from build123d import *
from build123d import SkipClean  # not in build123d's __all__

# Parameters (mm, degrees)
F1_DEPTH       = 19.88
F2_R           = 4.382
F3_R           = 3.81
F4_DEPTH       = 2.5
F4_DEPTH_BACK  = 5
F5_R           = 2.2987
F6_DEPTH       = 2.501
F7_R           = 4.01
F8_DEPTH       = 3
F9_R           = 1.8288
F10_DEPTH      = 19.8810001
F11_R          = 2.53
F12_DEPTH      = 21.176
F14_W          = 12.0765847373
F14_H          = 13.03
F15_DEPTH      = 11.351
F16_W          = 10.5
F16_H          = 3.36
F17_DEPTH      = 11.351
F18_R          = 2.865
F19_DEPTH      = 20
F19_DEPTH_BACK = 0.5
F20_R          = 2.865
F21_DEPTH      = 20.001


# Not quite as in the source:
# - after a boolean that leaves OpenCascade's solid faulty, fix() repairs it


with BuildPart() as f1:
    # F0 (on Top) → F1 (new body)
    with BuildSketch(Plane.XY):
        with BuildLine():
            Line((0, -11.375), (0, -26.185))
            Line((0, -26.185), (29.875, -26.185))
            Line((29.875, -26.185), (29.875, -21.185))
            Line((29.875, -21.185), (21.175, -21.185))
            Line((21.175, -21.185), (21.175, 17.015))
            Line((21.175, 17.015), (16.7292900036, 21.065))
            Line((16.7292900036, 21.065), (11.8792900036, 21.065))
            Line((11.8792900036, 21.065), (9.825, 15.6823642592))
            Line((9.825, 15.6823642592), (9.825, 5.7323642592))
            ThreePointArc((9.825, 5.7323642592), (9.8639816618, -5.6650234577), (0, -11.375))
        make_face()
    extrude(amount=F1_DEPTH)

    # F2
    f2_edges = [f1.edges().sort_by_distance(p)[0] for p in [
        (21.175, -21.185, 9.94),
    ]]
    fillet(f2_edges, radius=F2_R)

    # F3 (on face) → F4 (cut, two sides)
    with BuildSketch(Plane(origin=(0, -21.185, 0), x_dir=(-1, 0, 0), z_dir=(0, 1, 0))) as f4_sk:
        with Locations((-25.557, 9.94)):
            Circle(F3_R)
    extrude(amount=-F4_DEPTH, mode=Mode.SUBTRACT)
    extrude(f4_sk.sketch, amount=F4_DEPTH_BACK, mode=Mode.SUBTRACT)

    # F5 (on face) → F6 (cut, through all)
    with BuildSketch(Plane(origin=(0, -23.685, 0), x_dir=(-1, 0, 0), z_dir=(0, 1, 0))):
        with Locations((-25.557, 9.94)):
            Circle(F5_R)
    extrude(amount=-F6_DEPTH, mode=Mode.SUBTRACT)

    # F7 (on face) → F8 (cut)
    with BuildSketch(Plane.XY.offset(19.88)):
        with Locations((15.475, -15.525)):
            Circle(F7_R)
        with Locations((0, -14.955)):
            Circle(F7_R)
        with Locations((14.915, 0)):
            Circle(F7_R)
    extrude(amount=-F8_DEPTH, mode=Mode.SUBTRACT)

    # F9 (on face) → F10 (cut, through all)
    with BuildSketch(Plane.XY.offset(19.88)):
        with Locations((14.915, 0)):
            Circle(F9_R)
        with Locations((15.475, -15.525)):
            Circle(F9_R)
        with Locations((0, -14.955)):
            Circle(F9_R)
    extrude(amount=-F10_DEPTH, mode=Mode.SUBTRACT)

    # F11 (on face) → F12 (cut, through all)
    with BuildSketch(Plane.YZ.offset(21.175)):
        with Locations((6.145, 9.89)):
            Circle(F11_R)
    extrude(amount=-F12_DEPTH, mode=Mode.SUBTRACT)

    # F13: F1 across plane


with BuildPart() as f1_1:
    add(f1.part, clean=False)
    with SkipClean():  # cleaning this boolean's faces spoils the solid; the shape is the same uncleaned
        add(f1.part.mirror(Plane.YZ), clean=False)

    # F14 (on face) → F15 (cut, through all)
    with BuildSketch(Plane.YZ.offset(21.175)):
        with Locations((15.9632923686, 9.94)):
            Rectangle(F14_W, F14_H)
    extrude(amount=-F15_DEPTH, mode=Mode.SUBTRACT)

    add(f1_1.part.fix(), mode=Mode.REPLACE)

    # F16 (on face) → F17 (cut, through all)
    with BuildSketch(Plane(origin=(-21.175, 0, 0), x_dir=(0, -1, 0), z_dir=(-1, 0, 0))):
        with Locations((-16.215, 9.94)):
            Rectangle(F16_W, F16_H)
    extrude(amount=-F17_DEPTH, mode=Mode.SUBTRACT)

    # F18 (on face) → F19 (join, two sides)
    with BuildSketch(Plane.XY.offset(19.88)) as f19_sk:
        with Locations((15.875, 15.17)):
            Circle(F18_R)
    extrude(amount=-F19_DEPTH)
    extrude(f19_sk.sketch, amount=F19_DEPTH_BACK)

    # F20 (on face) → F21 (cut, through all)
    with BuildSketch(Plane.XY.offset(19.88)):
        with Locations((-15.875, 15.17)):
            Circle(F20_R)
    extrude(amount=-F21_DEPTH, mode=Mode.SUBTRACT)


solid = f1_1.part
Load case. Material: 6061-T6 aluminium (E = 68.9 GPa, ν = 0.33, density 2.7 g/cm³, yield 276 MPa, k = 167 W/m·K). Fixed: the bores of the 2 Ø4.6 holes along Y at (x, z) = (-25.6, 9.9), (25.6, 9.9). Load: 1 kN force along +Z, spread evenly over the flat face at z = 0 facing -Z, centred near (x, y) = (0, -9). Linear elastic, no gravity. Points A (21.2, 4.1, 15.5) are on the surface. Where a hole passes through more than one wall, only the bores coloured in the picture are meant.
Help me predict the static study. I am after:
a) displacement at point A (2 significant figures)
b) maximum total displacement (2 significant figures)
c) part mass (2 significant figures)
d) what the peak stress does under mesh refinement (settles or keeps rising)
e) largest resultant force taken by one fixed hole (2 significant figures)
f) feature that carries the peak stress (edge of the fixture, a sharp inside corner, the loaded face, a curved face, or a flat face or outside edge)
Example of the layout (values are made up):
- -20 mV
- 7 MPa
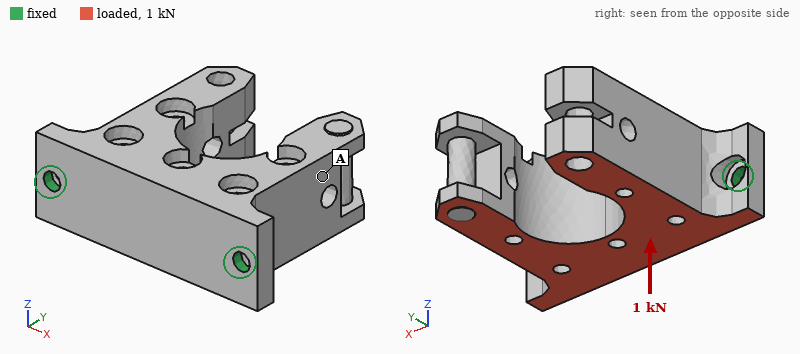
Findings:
- 0.14 mm
- 0.23 mm
- 66 g
- keeps rising
- 500 N
- edge of the fixture
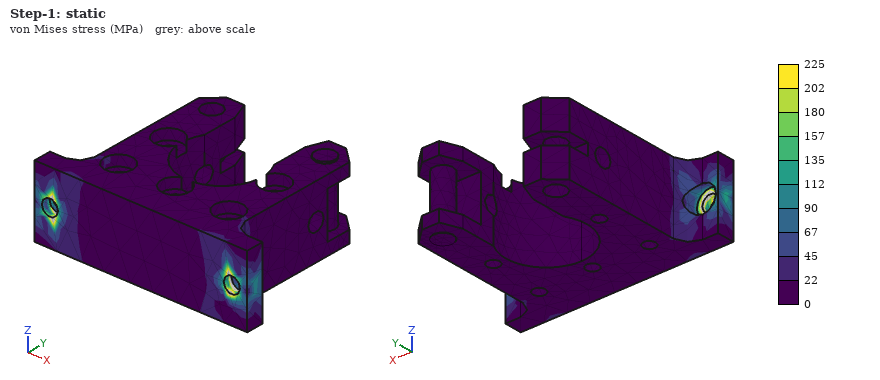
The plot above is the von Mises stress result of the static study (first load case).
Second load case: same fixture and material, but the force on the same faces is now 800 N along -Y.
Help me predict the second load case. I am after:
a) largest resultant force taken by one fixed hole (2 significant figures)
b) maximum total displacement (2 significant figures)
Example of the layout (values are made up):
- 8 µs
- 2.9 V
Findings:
- 480 N
- 0.11 mm
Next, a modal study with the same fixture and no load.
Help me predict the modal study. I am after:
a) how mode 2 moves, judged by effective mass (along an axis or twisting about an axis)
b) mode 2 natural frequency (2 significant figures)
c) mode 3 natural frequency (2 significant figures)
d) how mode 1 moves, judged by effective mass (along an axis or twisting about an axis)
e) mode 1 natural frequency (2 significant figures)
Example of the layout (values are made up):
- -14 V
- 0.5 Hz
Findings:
- twisting about Y
- 6300 Hz
- 6500 Hz
- along Z
- 1700 Hz
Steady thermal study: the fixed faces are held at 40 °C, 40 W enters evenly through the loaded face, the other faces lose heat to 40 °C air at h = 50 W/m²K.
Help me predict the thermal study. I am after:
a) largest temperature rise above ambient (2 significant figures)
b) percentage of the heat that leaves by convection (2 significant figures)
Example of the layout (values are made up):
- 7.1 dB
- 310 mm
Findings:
- 20 K
- 15 %
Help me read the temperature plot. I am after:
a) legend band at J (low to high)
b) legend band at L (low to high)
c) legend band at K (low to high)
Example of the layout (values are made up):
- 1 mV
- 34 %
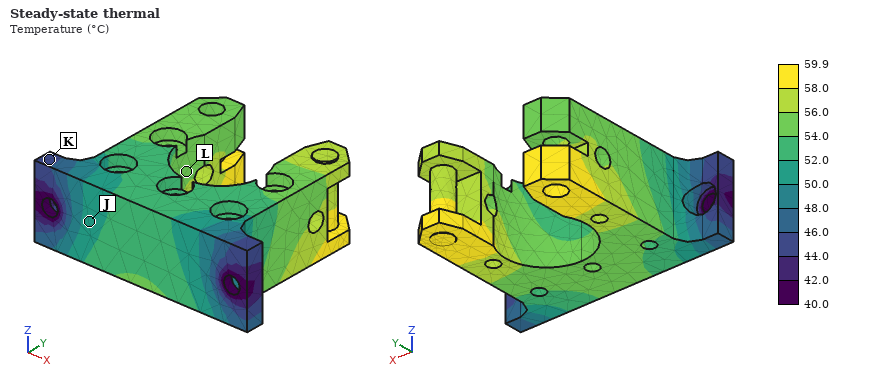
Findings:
- 50.0 to 52.0 °C
- 54.0 to 56.0 °C
- 44.0 to 46.0 °C
